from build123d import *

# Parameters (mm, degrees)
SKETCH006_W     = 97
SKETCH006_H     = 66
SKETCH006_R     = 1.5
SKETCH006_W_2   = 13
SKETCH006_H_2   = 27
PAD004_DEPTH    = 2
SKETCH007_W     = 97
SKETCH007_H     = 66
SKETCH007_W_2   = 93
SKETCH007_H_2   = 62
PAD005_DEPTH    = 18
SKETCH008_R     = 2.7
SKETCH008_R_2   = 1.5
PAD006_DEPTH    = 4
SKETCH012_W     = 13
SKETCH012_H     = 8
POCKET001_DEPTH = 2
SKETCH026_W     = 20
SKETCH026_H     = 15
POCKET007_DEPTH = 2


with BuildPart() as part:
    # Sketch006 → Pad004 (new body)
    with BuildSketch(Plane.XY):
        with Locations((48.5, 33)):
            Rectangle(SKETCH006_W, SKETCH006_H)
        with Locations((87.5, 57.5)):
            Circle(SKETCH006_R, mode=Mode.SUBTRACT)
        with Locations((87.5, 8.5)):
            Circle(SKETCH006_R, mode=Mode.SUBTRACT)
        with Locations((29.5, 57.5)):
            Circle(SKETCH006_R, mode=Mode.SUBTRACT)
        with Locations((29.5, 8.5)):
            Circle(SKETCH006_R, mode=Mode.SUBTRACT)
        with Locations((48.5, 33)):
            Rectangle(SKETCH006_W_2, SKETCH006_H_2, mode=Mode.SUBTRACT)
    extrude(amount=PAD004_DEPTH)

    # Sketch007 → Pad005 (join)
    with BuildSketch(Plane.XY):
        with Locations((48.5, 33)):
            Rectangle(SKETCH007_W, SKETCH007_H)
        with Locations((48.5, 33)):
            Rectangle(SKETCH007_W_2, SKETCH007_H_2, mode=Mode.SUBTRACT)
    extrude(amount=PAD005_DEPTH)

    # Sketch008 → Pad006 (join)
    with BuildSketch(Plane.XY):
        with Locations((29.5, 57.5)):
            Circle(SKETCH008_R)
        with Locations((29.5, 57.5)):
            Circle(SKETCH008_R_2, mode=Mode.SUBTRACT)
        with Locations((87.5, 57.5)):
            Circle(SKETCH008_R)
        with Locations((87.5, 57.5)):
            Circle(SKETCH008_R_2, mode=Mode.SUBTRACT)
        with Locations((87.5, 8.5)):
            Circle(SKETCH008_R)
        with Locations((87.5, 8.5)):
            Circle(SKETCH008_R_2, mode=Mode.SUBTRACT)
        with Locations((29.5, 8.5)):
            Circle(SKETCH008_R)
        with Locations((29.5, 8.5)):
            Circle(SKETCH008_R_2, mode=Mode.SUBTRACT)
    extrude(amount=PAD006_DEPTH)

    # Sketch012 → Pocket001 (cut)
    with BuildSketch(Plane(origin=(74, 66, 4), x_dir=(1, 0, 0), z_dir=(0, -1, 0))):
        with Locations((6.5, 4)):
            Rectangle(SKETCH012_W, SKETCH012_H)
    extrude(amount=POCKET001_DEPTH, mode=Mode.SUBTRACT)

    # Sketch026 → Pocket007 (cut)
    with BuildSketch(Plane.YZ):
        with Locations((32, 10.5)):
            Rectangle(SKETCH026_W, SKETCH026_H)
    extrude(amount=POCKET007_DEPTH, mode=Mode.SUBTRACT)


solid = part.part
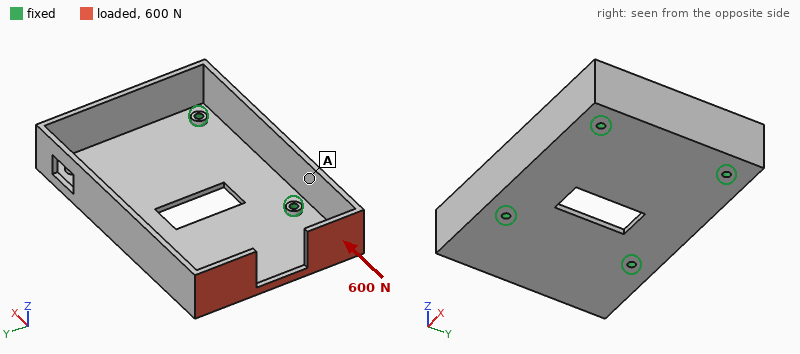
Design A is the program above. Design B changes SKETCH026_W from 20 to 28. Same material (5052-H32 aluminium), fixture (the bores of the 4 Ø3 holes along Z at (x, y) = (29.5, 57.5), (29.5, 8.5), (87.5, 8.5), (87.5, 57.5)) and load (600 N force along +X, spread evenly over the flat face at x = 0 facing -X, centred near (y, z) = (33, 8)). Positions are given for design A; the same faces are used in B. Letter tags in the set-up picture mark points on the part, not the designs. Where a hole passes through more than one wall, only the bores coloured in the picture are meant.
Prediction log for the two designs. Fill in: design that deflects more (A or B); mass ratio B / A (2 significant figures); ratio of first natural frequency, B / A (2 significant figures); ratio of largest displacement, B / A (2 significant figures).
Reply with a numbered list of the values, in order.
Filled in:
1. A
2. 0.99
3. 1.0
4. 0.81
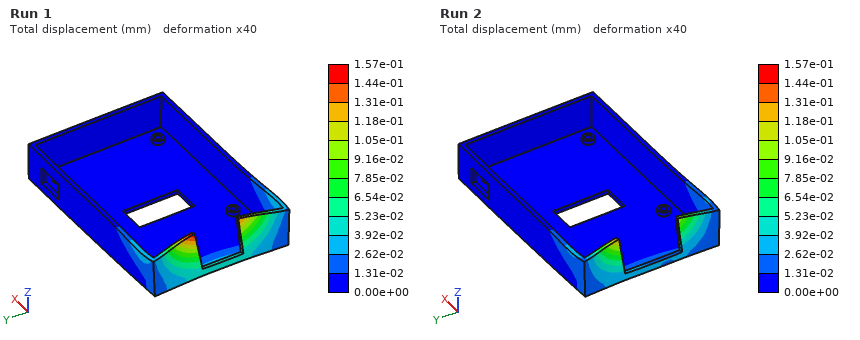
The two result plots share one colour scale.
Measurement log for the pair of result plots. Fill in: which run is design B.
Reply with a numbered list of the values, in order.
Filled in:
1. Run 2
